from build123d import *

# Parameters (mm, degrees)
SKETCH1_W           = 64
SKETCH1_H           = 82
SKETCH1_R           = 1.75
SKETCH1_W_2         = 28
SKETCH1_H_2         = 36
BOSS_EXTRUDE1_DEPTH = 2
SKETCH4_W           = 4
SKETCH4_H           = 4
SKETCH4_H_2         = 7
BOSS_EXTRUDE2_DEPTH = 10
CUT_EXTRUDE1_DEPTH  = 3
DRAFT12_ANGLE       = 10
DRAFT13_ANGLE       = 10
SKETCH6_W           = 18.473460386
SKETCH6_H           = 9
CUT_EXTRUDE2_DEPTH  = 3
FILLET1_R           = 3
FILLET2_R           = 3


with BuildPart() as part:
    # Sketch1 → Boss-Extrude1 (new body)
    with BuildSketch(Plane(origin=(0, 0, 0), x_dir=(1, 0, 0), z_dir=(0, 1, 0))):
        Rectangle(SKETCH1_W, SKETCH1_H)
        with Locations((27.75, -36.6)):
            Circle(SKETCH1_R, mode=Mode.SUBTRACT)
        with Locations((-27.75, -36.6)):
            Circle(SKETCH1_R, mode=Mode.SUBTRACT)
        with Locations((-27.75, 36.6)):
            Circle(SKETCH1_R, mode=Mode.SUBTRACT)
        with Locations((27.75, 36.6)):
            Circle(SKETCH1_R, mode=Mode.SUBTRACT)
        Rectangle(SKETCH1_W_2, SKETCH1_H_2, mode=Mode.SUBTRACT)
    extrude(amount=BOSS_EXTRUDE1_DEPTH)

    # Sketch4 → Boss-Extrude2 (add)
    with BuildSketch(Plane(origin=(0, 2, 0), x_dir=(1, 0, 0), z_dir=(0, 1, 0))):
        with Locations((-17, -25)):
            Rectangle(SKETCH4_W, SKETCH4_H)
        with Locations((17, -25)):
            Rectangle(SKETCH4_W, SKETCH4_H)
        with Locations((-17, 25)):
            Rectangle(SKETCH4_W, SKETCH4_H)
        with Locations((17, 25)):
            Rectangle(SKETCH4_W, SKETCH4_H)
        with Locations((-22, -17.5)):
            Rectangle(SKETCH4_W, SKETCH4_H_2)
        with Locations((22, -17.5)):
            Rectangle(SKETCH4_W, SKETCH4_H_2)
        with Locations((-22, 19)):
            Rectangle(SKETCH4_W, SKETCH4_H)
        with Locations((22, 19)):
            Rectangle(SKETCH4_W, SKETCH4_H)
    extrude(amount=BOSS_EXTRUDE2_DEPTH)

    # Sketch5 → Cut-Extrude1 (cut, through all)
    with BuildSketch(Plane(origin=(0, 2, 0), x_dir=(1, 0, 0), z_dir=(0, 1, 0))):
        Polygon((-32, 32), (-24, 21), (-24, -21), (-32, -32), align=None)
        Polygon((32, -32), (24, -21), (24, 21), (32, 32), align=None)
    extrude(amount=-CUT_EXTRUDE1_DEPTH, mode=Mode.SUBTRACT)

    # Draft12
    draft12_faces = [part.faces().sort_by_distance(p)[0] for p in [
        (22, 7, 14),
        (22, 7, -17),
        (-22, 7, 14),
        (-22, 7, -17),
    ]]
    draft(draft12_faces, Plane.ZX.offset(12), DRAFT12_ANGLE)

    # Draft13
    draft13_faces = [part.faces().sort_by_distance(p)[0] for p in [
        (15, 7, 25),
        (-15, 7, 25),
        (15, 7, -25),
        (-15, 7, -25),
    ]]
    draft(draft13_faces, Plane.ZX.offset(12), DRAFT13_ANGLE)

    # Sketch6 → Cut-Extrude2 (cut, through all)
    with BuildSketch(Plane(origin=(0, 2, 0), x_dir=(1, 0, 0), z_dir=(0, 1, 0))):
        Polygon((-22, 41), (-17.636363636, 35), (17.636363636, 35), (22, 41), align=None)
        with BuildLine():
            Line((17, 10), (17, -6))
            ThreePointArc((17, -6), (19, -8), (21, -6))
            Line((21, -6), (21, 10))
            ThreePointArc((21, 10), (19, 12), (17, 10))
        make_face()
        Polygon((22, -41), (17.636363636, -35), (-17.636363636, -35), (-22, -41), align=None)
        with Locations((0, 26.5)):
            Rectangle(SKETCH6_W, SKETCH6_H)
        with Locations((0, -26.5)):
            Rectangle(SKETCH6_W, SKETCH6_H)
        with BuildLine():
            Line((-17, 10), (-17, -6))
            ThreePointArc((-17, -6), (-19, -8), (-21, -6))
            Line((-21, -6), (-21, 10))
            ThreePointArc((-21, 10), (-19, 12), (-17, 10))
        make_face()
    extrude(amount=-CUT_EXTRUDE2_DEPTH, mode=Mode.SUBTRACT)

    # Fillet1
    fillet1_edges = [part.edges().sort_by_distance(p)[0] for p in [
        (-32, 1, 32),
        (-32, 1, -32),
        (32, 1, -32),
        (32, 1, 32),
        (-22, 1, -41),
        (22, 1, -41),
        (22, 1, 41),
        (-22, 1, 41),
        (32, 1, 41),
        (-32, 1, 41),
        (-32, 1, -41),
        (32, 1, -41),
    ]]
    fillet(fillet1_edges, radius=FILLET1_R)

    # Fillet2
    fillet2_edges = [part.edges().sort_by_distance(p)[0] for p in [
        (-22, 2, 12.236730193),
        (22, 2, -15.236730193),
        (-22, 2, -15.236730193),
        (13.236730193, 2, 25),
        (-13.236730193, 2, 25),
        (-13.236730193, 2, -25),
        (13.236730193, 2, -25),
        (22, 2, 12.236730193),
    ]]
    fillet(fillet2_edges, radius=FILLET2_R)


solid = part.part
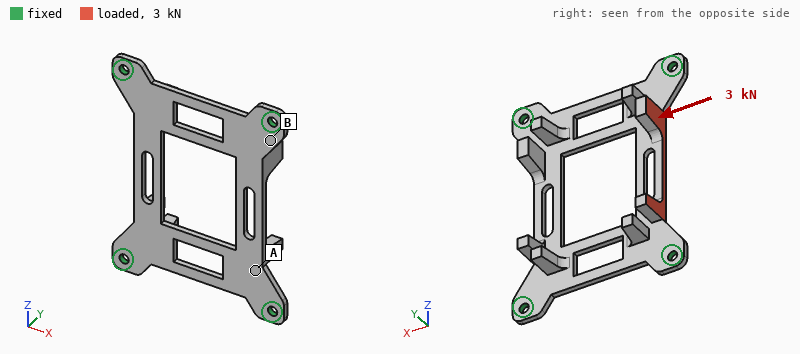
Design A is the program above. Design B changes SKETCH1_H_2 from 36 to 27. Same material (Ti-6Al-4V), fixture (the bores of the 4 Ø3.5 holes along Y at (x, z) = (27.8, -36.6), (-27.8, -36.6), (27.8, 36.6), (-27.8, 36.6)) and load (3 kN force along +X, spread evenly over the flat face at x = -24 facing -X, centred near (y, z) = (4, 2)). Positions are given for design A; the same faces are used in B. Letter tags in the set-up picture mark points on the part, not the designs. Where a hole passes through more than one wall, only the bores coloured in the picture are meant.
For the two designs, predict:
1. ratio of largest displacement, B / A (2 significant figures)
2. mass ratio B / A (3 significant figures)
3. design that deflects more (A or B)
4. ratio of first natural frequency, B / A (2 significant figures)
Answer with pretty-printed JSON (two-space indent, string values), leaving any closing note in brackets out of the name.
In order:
{
  "ratio of largest displacement, B / A": "0.84",
  "mass ratio B / A": "1.08",
  "design that deflects more": "A",
  "ratio of first natural frequency, B / A": "0.93"
}
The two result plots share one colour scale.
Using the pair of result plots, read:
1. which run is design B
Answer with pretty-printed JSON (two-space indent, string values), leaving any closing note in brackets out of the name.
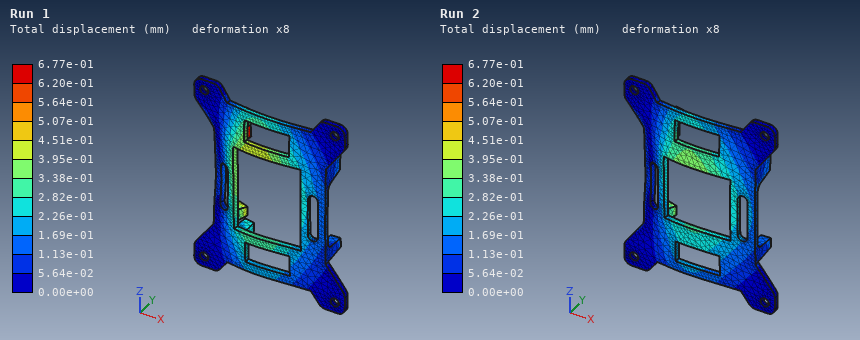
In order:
{
  "which run is design B": "Run 2"
}
